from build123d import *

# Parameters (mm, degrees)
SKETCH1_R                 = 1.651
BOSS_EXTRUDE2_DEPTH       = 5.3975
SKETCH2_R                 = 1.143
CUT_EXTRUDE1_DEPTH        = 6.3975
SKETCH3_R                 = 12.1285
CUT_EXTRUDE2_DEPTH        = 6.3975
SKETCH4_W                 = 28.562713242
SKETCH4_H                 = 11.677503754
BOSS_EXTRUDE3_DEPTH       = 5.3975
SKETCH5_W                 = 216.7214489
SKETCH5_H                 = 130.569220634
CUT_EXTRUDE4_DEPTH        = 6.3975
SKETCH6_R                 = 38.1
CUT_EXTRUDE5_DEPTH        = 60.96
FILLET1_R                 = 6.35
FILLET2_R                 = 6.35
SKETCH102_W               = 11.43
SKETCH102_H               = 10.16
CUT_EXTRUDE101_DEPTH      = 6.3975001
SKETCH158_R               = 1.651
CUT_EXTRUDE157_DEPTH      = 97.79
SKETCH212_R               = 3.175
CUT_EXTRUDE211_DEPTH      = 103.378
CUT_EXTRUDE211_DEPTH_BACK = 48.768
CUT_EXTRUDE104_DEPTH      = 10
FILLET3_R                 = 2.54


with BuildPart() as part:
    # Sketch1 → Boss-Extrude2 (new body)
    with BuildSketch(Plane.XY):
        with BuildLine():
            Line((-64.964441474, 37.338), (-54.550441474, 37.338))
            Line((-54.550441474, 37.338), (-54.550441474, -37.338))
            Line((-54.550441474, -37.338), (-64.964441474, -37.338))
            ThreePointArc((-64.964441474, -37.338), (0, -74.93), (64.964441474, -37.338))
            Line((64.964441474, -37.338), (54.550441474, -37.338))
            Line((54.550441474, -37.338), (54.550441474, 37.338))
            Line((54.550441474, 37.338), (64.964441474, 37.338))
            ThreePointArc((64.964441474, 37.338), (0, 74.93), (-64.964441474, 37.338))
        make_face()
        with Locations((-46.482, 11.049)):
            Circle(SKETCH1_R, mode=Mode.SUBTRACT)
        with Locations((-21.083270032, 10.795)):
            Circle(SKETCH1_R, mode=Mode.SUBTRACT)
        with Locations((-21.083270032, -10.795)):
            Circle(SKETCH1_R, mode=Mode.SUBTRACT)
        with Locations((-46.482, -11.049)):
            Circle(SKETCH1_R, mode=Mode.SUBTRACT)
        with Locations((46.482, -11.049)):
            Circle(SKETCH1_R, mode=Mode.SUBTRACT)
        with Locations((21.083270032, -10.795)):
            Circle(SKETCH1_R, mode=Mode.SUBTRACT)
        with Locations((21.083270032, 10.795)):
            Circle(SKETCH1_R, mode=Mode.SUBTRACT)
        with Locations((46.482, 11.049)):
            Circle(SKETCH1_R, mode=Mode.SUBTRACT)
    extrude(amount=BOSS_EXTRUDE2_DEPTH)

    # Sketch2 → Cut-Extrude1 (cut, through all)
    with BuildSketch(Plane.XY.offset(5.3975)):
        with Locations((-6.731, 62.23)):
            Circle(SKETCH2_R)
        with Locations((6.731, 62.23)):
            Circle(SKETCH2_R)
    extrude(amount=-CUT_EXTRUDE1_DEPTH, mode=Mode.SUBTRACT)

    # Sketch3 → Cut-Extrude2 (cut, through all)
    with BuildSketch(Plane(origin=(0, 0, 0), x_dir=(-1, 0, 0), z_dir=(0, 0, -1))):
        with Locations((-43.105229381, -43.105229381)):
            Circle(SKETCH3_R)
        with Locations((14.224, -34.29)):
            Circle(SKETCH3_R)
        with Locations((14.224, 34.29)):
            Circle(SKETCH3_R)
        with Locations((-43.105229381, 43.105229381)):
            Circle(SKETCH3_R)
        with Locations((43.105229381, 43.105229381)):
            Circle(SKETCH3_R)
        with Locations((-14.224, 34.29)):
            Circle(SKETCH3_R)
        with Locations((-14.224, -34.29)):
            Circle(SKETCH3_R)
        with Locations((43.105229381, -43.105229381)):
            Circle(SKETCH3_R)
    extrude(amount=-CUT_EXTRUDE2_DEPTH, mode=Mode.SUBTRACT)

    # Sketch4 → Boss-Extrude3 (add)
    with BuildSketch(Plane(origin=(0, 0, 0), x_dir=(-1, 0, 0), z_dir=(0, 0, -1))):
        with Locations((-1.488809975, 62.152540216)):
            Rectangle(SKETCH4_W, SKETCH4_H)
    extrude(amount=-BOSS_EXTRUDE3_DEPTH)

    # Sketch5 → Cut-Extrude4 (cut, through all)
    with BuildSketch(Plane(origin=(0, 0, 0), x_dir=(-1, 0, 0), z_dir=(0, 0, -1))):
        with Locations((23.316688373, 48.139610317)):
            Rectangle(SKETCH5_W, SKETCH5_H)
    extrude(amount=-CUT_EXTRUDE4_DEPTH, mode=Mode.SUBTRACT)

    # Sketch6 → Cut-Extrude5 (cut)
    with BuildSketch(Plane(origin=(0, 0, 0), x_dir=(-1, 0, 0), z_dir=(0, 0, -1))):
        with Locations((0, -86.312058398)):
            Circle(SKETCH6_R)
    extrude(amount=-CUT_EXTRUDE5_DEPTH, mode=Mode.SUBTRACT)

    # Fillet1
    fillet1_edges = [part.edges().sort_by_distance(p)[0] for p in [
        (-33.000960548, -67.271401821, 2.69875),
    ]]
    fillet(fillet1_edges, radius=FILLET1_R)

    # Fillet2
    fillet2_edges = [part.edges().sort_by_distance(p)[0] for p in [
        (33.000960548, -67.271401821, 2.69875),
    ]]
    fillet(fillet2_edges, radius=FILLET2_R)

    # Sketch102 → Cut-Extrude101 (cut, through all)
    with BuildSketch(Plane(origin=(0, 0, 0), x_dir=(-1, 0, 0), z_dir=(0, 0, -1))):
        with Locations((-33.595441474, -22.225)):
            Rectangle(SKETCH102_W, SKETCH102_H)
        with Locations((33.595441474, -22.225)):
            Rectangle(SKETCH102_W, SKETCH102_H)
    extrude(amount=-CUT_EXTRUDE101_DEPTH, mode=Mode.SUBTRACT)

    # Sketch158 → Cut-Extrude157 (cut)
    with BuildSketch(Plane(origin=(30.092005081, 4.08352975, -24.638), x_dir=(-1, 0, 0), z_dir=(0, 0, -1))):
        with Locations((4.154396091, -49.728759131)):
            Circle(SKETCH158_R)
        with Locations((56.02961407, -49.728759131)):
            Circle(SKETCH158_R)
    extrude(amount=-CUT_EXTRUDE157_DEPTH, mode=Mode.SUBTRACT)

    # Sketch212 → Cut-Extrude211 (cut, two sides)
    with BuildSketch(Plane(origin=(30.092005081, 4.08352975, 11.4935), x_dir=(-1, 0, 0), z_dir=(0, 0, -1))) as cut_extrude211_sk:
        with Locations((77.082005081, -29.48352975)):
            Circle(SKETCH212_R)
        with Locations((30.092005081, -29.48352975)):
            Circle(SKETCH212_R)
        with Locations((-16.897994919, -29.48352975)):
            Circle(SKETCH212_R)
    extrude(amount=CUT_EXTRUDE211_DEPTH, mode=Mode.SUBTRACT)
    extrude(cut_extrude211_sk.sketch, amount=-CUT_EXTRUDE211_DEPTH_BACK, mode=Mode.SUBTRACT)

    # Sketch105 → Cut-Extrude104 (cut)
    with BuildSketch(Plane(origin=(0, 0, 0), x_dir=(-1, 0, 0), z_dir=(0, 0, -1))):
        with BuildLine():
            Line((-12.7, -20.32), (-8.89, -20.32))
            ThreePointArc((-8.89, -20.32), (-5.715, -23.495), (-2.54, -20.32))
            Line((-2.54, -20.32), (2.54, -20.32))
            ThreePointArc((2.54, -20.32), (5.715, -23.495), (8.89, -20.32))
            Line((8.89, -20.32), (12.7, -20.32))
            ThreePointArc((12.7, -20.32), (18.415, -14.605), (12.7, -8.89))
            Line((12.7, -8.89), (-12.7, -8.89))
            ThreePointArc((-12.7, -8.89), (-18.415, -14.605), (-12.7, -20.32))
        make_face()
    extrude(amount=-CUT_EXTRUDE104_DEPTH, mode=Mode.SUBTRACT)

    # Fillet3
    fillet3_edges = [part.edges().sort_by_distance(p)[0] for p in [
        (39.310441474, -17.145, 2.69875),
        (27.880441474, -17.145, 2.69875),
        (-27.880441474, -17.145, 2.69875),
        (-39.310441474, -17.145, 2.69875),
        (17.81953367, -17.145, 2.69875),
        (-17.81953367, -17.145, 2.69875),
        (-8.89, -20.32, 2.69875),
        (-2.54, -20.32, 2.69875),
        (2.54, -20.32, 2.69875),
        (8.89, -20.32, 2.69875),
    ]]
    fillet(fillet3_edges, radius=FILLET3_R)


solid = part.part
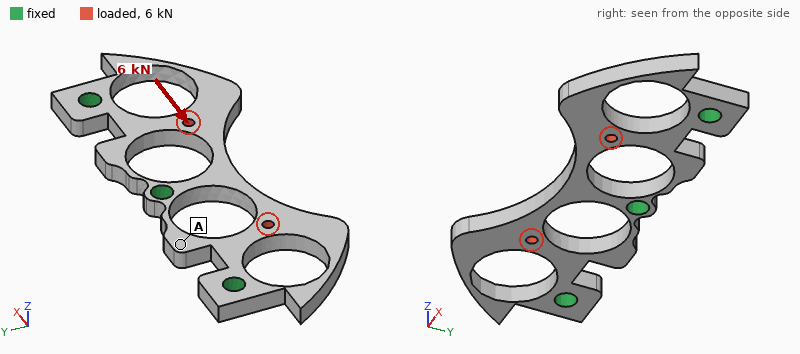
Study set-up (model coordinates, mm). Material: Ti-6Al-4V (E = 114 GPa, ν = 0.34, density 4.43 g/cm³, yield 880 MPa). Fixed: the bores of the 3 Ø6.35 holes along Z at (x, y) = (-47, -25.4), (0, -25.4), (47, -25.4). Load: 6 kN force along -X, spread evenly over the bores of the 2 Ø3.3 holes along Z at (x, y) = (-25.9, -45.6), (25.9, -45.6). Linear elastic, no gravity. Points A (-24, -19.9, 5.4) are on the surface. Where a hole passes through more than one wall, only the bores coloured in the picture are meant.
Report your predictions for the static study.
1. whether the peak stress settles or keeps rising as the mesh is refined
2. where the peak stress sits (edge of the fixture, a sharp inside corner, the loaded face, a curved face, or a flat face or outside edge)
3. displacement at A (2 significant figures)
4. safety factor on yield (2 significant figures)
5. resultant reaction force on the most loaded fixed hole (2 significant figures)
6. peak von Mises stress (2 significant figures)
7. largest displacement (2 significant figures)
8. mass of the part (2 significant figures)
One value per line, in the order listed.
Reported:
settles
a curved face
36 µm
2.7
2.5 kN
330 MPa
86 µm
50 g
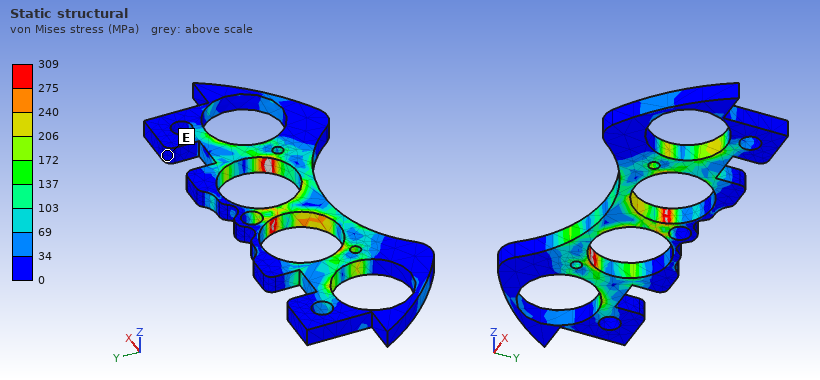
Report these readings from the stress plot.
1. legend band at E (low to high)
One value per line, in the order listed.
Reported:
0 to 34 MPa
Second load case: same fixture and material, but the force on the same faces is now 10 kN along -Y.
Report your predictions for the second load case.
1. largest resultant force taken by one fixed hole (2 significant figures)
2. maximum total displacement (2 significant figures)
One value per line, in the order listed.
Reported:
4.3 kN
0.11 mm
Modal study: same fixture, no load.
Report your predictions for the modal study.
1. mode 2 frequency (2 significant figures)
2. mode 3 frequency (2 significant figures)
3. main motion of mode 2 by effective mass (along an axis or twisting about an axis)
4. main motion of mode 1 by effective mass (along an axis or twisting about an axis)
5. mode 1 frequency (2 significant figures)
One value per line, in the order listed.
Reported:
2300 Hz
5800 Hz
twisting about Y
along Z
2000 Hz
